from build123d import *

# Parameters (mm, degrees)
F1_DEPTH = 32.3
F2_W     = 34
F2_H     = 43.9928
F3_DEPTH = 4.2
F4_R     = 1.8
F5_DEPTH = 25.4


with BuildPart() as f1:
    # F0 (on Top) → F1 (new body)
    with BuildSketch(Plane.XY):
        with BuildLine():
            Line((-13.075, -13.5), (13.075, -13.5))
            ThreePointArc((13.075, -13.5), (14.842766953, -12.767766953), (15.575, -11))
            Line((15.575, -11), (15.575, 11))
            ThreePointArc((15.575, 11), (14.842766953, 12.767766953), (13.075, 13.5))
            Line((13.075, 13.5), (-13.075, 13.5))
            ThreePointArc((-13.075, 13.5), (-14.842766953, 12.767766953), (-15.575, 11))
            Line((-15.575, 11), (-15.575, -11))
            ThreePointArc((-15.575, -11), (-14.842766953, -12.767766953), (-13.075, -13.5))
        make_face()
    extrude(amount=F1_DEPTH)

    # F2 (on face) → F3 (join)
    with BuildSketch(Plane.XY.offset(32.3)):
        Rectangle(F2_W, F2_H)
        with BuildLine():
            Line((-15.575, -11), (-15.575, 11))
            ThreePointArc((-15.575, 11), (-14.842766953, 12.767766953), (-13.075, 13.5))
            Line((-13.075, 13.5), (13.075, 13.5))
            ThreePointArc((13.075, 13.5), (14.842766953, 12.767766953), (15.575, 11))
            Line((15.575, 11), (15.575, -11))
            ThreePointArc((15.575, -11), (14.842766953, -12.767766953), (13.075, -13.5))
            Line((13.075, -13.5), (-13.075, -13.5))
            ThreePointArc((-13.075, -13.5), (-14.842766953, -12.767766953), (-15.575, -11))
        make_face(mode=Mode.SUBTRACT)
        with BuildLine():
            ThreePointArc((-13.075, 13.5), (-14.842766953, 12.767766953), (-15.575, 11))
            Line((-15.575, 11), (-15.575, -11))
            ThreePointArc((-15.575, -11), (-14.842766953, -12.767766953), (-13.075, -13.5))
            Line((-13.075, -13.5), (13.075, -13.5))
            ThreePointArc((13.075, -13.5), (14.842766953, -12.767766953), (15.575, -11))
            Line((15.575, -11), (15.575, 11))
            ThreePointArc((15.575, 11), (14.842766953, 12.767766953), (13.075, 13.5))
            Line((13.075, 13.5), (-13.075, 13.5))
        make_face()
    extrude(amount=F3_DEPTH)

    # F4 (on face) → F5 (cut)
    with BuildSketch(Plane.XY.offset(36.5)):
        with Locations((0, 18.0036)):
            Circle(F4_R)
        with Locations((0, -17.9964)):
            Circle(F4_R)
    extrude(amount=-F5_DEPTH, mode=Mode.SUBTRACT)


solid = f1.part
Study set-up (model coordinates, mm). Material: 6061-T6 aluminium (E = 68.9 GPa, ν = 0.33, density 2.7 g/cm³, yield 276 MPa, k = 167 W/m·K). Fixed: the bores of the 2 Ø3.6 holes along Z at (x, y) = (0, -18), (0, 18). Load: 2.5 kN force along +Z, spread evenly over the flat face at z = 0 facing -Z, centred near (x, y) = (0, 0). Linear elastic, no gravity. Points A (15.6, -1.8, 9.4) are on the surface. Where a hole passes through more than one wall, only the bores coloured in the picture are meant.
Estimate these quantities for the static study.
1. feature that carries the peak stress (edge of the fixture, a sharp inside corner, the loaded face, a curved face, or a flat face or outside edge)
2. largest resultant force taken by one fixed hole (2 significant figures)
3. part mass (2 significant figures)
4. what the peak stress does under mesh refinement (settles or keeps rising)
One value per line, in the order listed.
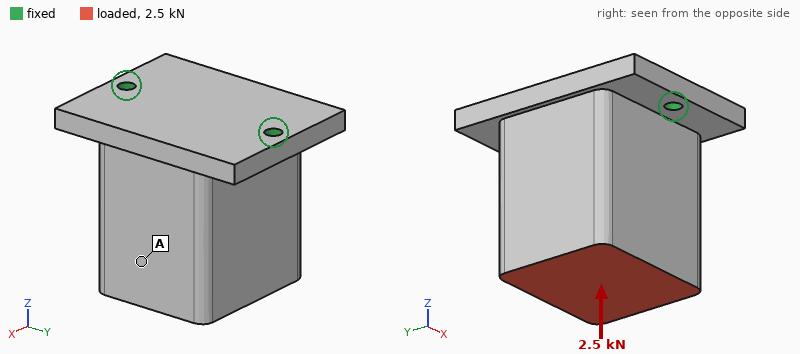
edge of the fixture
1.3 kN
90 g
keeps rising
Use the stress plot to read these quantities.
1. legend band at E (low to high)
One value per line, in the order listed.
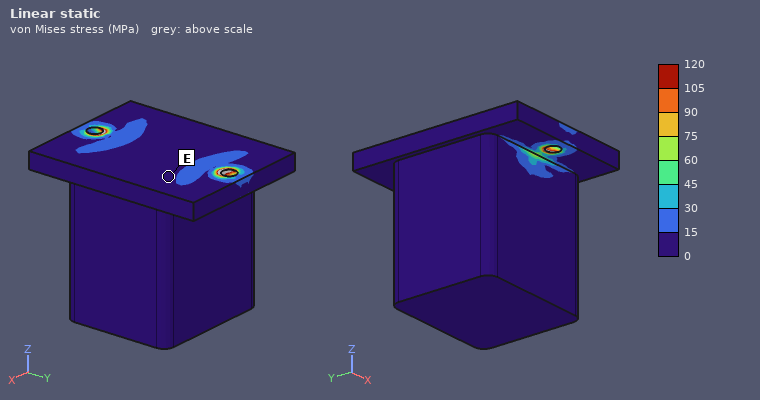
0 to 15 MPa
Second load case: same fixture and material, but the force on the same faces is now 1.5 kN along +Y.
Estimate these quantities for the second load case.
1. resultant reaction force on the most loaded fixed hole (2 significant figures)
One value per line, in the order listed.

1.8 kN
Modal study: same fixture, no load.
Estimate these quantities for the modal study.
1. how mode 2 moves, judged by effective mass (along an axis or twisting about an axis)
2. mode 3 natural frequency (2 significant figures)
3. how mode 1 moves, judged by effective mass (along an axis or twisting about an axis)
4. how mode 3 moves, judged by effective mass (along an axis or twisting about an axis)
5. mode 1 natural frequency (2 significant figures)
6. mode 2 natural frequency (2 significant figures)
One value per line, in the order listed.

along Y
8200 Hz
along X
along Z
1800 Hz
6100 Hz
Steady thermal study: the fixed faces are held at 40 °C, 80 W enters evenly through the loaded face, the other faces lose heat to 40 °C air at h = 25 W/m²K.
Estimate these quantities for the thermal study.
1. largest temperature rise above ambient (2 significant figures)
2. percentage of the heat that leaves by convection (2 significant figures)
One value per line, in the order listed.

41 K
5.1 %
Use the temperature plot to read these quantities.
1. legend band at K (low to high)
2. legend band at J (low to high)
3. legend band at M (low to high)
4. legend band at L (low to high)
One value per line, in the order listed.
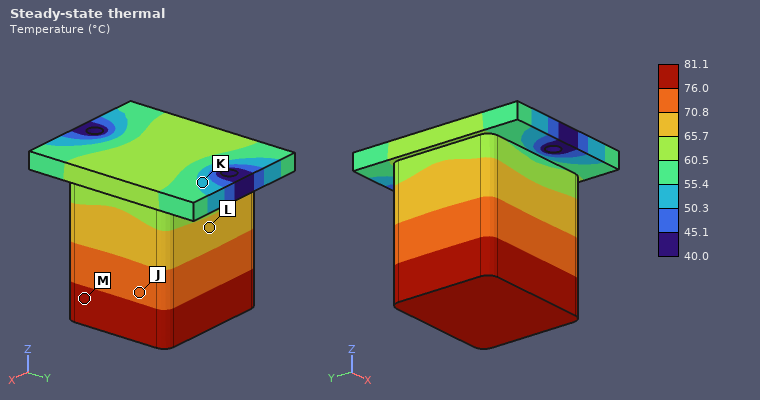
50.3 to 55.4 °C
70.8 to 76.0 °C
76.0 to 81.1 °C
65.7 to 70.8 °C
